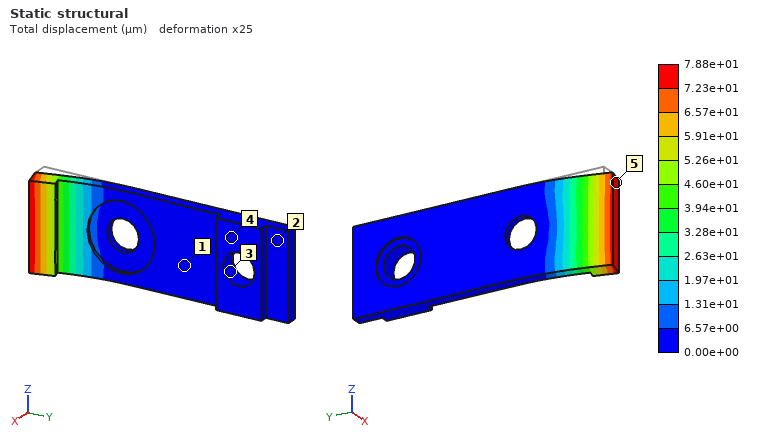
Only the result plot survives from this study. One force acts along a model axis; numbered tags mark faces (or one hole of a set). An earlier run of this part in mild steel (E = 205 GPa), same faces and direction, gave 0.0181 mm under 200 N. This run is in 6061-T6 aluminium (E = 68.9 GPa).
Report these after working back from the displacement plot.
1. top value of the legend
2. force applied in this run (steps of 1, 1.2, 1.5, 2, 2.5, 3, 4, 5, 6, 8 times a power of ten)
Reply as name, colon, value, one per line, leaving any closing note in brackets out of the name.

top value of the legend: 7.88e+01 µm
force applied in this run: 300 N
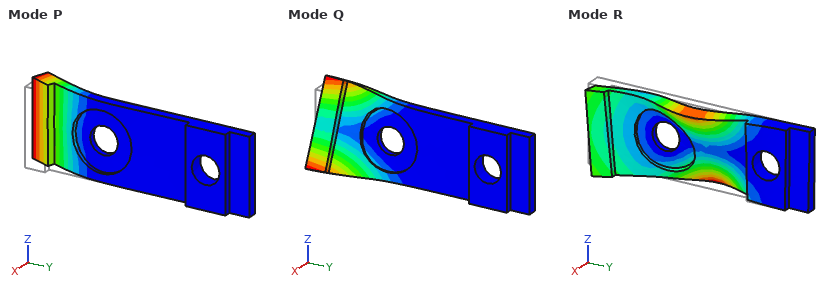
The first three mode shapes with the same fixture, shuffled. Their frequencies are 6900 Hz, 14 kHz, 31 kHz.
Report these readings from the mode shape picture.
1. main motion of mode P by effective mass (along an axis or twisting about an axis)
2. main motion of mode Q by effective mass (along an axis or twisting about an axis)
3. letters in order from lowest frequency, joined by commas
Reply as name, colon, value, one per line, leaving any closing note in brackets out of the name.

main motion of mode P by effective mass: along X
main motion of mode Q by effective mass: twisting about Y
letters in order from lowest frequency, joined by commas: P, Q, R
